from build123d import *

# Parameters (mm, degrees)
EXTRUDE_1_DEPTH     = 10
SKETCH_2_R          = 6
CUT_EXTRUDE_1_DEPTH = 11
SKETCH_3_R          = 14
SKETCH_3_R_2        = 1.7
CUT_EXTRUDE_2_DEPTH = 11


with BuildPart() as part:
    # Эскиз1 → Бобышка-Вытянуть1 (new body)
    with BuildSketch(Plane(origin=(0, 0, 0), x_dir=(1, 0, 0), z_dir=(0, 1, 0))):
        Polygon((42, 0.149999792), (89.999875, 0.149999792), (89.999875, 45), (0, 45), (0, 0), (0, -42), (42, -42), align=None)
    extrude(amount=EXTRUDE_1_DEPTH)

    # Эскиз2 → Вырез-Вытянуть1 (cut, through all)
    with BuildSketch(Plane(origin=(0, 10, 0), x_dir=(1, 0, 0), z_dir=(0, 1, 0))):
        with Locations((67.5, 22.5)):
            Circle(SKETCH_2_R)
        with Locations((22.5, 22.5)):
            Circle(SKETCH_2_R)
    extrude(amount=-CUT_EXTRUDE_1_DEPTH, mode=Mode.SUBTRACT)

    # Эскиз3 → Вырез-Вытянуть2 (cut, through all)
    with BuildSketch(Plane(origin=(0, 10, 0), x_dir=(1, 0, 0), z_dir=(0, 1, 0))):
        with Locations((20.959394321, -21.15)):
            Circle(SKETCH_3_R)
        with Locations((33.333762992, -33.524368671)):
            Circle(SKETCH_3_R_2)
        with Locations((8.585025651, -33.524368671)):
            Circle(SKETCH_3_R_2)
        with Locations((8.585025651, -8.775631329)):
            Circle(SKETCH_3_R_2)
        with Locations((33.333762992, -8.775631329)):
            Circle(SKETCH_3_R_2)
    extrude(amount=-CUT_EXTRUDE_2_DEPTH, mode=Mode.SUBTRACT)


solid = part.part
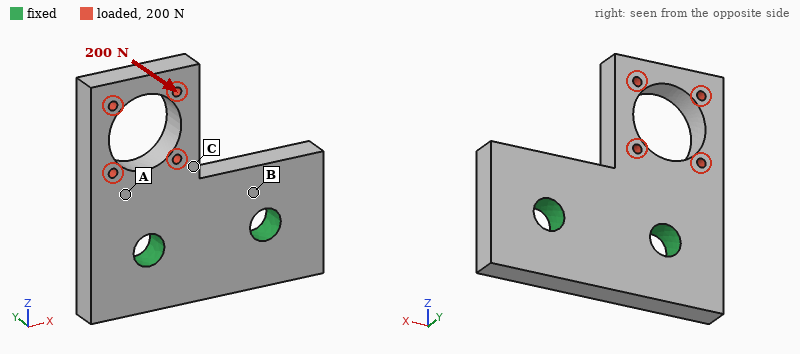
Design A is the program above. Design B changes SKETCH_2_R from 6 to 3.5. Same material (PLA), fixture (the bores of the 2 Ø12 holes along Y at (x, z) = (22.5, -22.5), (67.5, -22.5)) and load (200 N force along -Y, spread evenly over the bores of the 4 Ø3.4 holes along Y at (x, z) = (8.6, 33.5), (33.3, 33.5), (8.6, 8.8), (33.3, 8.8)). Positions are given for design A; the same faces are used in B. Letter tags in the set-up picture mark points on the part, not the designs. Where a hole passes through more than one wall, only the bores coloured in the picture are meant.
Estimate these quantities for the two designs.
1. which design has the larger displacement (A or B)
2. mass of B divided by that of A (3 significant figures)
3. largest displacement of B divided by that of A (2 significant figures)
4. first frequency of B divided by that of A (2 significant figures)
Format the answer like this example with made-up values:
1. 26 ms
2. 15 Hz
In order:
1. B
2. 1.03
3. 1.2
4. 0.92
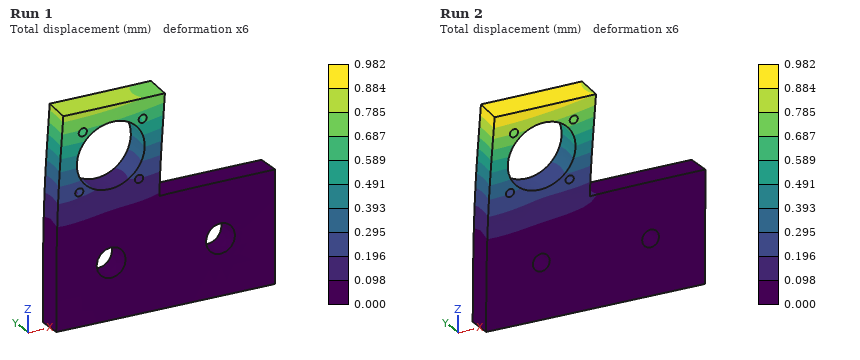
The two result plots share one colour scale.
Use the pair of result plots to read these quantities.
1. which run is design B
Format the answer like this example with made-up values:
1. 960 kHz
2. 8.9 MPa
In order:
1. Run 2
